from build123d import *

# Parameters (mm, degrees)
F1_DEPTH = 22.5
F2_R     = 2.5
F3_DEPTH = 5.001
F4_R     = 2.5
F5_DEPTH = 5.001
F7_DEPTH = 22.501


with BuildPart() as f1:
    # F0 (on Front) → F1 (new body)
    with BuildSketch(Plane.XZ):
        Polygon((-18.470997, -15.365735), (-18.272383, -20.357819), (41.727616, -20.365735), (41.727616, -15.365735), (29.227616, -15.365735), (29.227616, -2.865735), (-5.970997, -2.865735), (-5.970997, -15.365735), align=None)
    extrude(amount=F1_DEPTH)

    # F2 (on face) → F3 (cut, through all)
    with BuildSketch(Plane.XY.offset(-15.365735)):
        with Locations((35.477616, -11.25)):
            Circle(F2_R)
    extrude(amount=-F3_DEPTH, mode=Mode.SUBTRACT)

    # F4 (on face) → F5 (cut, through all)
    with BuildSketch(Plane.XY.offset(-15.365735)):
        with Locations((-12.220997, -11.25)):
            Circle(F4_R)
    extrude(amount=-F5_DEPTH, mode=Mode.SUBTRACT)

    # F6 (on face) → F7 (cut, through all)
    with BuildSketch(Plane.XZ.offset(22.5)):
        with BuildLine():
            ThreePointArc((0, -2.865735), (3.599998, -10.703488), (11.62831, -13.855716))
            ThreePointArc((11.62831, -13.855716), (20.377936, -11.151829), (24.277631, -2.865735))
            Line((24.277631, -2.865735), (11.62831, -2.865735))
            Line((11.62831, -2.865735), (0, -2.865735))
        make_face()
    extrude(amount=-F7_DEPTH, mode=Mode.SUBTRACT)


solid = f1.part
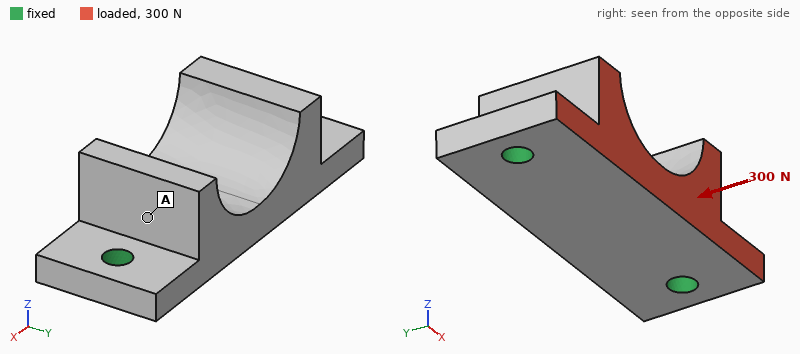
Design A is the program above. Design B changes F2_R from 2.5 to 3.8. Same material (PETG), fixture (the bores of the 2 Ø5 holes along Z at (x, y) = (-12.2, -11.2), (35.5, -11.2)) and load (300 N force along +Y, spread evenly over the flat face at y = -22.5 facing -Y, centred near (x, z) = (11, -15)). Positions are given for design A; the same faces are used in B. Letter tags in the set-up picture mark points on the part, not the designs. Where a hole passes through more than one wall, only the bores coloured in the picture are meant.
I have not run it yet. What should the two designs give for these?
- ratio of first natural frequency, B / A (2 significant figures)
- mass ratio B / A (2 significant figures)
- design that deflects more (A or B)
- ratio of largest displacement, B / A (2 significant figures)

1.1
0.99
A
0.88
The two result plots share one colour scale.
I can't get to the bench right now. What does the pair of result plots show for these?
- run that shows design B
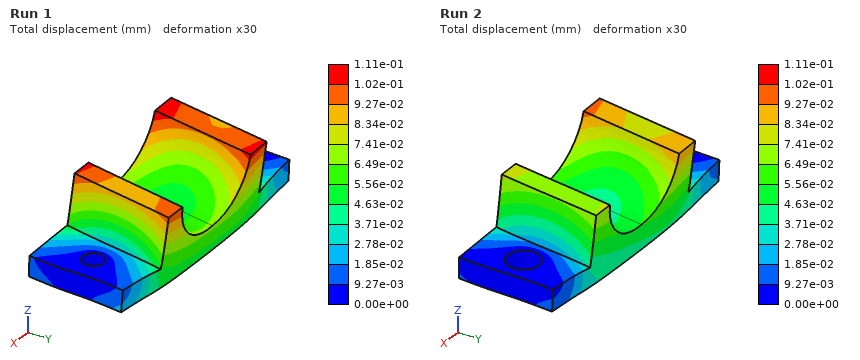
Run 2
